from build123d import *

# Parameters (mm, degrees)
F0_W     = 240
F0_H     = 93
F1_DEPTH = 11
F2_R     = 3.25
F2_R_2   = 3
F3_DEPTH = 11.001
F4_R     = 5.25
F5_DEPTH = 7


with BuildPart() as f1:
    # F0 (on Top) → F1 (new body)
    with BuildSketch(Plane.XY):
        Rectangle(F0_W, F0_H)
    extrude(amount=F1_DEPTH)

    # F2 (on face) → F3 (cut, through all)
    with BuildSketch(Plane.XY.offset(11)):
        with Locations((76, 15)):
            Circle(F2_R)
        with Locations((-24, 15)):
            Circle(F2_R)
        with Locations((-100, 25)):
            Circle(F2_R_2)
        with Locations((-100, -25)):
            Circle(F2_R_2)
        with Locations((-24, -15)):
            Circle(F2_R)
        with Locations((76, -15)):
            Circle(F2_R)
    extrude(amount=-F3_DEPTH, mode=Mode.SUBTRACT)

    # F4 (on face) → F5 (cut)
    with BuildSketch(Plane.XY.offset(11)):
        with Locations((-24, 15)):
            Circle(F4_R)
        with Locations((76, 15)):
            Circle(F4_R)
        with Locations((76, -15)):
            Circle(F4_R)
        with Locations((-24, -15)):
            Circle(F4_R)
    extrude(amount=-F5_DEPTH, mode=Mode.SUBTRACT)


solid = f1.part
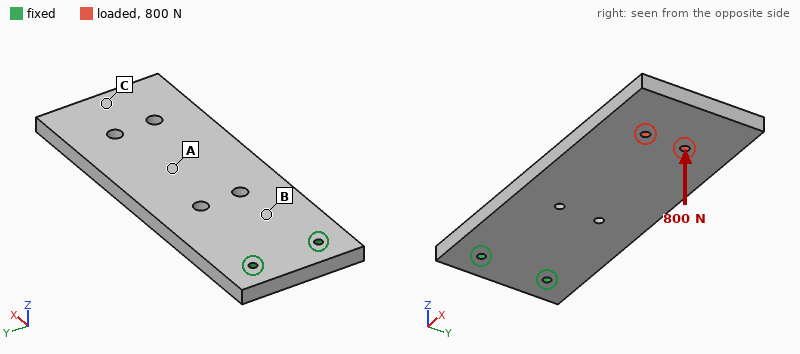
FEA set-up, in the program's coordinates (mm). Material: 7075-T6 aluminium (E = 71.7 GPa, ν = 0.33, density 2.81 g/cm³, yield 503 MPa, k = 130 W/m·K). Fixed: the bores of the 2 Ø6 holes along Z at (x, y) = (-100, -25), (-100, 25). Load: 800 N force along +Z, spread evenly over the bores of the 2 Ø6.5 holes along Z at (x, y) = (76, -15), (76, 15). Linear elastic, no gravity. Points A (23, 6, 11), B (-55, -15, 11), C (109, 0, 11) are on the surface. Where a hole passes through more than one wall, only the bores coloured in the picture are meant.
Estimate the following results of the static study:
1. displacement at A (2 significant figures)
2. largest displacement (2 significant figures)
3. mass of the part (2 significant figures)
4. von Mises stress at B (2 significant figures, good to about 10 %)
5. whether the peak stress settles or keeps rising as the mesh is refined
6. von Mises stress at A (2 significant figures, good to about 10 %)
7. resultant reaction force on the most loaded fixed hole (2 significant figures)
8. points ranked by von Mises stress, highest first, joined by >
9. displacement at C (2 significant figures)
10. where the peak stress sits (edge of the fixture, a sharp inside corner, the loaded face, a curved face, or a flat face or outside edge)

1.2 mm
2.9 mm
680 g
52 MPa
keeps rising
23 MPa
400 N
B > A > C
2.7 mm
edge of the fixture
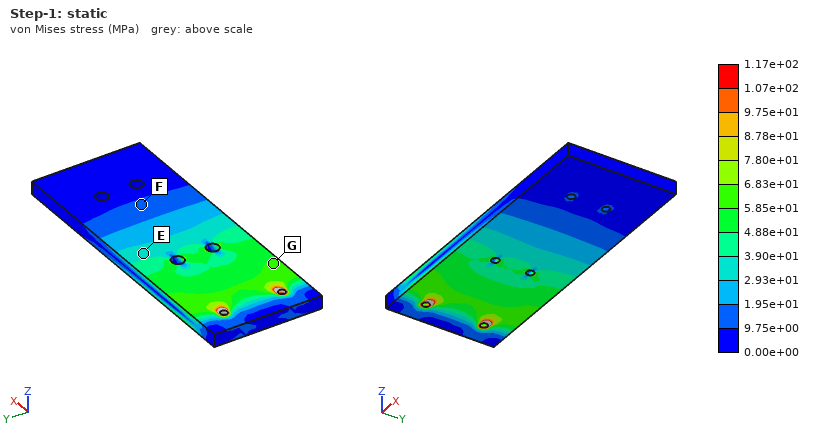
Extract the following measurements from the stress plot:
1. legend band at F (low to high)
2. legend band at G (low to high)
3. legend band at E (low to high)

9.75e+00 to 1.95e+01 MPa
5.85e+01 to 6.83e+01 MPa
2.93e+01 to 3.90e+01 MPa
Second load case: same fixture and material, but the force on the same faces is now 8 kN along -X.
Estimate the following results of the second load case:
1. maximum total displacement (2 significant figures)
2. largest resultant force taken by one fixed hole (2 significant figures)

0.92 mm
4.0 kN
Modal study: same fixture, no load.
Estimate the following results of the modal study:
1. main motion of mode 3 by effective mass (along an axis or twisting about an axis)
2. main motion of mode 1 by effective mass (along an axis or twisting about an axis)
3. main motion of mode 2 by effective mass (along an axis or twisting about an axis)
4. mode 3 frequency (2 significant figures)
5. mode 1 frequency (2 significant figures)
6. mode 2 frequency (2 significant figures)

along Z
along Z
twisting about X
1100 Hz
180 Hz
860 Hz
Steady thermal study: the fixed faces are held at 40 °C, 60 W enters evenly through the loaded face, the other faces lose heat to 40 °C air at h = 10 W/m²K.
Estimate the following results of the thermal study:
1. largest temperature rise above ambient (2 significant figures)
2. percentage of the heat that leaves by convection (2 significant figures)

74 K
31 %
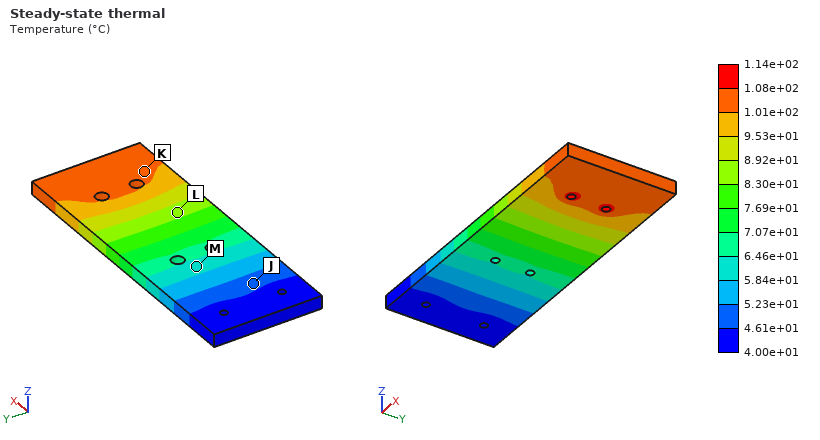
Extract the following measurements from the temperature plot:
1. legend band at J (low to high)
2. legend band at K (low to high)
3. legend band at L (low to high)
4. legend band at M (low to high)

4.61e+01 to 5.23e+01 °C
1.01e+02 to 1.08e+02 °C
8.30e+01 to 8.92e+01 °C
5.84e+01 to 6.46e+01 °C
